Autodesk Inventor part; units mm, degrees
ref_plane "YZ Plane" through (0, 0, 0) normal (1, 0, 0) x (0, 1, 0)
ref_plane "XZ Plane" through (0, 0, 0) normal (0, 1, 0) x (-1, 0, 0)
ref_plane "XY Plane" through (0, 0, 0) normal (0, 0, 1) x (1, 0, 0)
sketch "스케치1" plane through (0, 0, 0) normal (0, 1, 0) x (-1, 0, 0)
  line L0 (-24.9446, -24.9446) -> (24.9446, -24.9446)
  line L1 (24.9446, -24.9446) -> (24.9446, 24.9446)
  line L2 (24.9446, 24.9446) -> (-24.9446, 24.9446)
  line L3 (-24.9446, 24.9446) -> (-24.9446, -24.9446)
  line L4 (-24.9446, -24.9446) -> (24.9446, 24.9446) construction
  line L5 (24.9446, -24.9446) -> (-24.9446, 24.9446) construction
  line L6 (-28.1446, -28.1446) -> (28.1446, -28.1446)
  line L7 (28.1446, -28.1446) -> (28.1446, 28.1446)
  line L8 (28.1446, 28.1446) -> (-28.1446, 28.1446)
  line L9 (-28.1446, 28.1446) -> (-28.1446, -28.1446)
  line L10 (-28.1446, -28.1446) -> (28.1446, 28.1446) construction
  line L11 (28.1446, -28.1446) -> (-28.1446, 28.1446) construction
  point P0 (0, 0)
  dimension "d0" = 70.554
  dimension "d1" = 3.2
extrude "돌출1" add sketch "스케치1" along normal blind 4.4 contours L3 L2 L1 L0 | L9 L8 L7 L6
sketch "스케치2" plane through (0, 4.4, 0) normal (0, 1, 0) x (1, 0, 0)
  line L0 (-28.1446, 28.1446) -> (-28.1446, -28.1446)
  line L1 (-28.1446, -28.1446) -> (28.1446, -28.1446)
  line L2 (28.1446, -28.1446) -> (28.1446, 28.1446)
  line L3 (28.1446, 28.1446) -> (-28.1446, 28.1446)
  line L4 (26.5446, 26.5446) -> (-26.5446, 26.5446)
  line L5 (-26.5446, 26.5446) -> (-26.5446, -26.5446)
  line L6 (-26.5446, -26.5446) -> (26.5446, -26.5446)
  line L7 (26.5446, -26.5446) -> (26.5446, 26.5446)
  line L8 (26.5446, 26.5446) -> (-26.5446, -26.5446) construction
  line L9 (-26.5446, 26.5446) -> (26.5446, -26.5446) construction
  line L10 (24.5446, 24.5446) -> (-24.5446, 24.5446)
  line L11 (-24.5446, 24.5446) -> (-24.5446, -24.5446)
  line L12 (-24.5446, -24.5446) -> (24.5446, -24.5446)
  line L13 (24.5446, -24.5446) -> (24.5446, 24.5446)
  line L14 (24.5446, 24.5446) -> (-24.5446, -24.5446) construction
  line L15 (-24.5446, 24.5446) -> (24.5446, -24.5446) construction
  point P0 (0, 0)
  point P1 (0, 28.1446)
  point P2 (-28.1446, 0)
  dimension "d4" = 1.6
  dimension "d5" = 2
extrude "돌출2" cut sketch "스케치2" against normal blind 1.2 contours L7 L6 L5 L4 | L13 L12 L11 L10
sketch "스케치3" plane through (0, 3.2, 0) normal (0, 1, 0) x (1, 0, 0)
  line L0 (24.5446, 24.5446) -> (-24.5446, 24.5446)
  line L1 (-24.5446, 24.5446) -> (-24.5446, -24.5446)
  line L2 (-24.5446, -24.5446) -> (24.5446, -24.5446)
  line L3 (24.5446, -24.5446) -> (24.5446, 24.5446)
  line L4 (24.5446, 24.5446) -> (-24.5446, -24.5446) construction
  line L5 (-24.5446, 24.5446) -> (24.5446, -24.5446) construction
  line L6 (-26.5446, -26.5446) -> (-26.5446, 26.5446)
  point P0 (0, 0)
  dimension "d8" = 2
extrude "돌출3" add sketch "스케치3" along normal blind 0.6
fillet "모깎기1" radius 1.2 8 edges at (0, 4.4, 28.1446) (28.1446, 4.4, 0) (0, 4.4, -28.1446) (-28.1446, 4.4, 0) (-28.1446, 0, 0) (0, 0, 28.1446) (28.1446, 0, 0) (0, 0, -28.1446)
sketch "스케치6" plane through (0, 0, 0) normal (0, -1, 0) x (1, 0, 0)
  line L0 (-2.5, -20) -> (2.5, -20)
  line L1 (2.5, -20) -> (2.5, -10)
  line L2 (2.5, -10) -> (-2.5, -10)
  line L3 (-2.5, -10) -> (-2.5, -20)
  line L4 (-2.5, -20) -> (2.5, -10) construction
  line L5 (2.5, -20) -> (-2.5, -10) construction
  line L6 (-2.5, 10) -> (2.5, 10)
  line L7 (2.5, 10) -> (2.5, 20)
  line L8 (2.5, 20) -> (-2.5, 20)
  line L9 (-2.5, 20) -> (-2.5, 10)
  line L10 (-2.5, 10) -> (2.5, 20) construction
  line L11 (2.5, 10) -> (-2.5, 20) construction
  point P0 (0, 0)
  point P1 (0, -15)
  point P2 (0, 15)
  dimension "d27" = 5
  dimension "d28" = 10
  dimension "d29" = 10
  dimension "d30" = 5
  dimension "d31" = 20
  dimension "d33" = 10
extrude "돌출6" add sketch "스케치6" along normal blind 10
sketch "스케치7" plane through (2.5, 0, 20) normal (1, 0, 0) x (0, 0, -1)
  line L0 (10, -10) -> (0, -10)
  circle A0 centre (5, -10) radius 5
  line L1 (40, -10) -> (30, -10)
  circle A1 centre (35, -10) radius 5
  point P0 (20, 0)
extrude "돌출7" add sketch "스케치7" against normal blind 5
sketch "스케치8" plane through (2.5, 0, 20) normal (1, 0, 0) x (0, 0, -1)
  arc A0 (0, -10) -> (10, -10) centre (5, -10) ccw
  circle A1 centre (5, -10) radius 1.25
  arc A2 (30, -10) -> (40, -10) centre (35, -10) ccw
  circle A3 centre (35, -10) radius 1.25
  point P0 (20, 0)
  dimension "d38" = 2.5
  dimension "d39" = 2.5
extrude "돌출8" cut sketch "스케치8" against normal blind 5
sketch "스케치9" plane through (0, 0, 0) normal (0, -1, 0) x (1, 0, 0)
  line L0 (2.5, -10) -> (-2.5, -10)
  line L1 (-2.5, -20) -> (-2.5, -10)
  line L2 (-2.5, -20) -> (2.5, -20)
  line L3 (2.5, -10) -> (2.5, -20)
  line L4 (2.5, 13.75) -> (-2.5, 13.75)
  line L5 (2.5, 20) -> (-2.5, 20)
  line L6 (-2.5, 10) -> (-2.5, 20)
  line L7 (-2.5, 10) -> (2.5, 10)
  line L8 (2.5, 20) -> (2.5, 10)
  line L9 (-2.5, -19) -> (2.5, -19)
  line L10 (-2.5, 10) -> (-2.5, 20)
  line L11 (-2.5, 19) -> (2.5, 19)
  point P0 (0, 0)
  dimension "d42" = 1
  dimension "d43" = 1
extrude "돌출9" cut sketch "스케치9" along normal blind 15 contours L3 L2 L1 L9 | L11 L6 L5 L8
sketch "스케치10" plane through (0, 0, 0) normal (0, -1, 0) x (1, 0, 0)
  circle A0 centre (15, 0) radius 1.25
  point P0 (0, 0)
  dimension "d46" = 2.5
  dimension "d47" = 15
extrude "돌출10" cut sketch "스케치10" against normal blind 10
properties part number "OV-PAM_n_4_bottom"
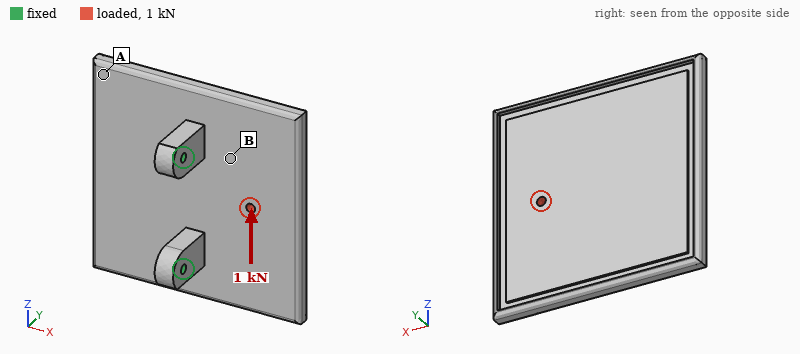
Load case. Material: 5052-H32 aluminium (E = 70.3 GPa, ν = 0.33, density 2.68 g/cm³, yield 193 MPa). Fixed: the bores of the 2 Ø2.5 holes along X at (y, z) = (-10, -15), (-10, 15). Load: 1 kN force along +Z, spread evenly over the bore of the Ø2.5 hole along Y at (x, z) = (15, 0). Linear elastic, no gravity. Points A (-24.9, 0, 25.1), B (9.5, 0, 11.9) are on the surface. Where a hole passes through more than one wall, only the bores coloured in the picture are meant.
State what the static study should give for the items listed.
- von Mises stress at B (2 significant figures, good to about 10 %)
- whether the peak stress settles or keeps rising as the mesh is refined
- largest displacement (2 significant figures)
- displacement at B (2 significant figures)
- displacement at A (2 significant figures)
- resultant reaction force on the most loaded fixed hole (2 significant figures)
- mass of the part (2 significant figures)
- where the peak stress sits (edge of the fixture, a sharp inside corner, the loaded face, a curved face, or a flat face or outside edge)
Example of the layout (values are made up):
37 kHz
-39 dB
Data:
29 MPa
keeps rising
79 µm
38 µm
54 µm
700 N
35 g
edge of the fixture
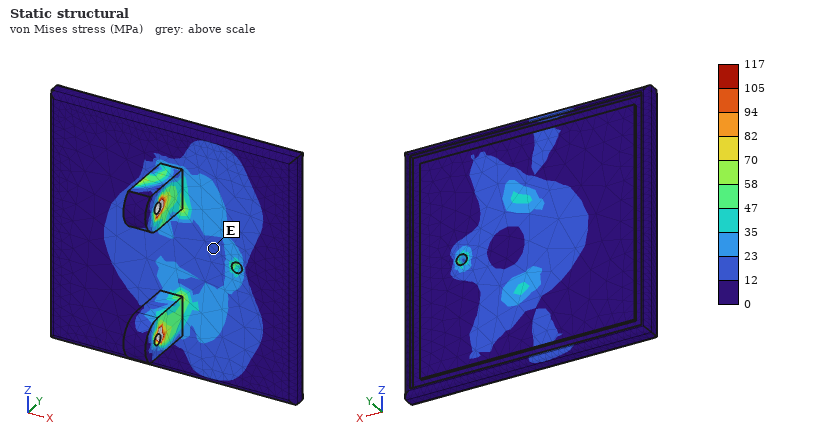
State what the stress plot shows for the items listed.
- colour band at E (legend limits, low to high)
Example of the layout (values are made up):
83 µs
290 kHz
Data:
12 to 23 MPa
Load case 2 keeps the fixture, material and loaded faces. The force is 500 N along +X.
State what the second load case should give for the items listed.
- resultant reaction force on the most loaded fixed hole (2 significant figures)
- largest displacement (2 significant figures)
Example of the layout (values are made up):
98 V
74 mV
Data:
250 N
82 µm
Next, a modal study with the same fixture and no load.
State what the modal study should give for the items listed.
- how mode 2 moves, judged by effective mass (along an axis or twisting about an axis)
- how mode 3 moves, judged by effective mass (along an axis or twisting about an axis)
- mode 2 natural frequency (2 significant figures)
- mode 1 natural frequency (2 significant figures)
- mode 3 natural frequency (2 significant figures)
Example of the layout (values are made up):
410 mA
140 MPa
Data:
twisting about Y
along Y
3400 Hz
1600 Hz
4200 Hz
